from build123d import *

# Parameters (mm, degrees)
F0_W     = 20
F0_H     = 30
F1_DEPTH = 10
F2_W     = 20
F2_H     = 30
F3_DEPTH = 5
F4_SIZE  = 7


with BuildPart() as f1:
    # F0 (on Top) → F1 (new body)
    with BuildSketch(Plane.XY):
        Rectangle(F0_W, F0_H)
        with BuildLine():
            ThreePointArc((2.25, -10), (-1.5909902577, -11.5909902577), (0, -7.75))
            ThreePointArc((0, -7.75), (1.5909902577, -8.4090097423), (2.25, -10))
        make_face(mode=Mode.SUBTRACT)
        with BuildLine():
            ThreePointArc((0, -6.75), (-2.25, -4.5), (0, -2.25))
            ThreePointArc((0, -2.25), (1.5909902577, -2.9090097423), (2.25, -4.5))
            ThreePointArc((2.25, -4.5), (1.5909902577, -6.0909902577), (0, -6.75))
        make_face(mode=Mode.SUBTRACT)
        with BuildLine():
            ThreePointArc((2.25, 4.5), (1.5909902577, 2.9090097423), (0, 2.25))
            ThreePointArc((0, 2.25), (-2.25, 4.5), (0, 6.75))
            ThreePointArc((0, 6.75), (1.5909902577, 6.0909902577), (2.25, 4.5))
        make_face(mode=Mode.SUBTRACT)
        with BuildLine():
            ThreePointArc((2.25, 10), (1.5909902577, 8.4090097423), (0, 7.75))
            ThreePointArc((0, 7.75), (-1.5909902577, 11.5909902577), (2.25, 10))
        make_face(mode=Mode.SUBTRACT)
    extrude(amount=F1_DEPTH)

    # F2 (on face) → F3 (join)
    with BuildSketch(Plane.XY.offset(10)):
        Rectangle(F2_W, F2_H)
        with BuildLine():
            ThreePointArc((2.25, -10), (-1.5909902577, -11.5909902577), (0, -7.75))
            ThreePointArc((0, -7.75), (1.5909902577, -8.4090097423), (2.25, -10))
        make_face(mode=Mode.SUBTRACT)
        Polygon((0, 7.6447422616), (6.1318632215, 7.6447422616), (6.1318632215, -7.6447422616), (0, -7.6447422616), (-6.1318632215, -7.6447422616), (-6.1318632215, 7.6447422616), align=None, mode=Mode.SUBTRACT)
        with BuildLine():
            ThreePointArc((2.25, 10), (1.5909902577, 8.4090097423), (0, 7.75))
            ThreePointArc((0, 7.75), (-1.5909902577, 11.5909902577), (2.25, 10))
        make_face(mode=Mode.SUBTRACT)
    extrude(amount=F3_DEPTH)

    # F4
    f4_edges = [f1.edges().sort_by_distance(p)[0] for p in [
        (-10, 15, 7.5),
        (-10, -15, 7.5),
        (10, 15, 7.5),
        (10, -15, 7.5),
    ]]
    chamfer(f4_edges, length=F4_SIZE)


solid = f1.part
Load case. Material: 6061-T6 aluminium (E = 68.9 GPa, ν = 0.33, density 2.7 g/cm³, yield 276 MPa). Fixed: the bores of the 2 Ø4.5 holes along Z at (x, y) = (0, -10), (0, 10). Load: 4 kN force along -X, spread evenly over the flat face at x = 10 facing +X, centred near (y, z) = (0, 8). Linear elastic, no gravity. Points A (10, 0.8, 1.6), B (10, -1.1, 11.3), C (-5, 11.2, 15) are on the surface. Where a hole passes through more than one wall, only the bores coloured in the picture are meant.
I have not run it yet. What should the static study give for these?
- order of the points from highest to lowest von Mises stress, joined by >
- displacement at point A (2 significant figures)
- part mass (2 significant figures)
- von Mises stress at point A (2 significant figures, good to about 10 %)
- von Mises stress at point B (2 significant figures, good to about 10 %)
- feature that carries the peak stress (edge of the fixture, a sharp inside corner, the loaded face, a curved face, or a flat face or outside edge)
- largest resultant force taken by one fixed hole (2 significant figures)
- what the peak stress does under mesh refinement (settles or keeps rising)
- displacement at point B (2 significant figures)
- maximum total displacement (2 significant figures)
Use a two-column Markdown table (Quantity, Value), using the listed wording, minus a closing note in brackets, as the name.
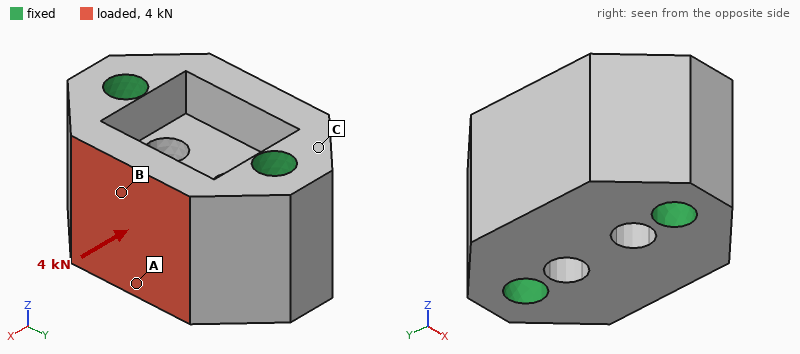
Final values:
| Quantity | Value |
|---|---|
| order of the points from highest to lowest von Mises stress, joined by > | B > A > C |
| displacement at point A | 4.0 µm |
| part mass | 16 g |
| von Mises stress at point A | 23 MPa |
| von Mises stress at point B | 47 MPa |
| feature that carries the peak stress | a sharp inside corner |
| largest resultant force taken by one fixed hole | 2.1 kN |
| what the peak stress does under mesh refinement | keeps rising |
| displacement at point B | 11 µm |
| maximum total displacement | 17 µm |
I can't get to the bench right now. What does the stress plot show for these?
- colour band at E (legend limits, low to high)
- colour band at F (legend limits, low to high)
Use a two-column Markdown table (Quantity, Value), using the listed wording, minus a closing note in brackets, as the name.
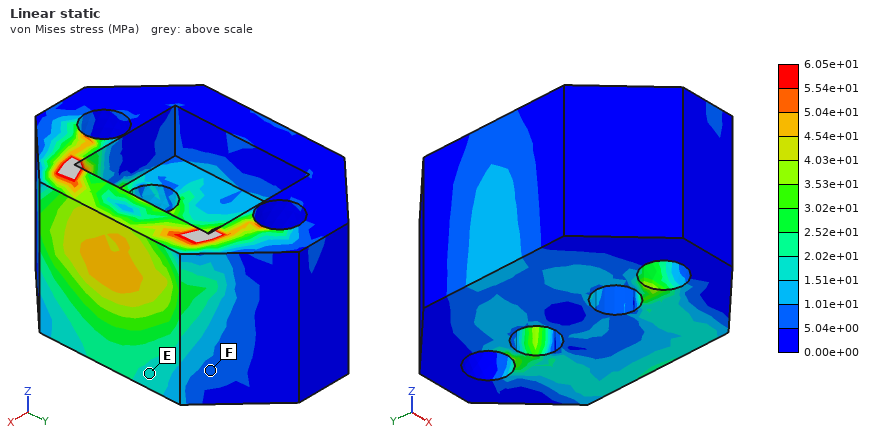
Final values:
| Quantity | Value |
|---|---|
| colour band at E | 1.51e+01 to 2.02e+01 MPa |
| colour band at F | 5.04e+00 to 1.01e+01 MPa |
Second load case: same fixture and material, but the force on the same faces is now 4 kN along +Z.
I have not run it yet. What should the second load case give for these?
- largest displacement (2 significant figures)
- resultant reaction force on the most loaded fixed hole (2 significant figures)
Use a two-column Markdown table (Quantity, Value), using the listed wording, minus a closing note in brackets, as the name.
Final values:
| Quantity | Value |
|---|---|
| largest displacement | 27 µm |
| resultant reaction force on the most loaded fixed hole | 2.0 kN |
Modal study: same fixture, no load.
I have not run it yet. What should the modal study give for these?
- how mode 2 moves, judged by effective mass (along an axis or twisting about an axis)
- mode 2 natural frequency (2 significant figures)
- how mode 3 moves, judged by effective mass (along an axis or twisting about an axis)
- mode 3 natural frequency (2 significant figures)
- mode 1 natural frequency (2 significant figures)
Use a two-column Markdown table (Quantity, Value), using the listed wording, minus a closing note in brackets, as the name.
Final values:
| Quantity | Value |
|---|---|
| how mode 2 moves, judged by effective mass | along Z |
| mode 2 natural frequency | 50 kHz |
| how mode 3 moves, judged by effective mass | along X |
| mode 3 natural frequency | 59 kHz |
| mode 1 natural frequency | 48 kHz |
